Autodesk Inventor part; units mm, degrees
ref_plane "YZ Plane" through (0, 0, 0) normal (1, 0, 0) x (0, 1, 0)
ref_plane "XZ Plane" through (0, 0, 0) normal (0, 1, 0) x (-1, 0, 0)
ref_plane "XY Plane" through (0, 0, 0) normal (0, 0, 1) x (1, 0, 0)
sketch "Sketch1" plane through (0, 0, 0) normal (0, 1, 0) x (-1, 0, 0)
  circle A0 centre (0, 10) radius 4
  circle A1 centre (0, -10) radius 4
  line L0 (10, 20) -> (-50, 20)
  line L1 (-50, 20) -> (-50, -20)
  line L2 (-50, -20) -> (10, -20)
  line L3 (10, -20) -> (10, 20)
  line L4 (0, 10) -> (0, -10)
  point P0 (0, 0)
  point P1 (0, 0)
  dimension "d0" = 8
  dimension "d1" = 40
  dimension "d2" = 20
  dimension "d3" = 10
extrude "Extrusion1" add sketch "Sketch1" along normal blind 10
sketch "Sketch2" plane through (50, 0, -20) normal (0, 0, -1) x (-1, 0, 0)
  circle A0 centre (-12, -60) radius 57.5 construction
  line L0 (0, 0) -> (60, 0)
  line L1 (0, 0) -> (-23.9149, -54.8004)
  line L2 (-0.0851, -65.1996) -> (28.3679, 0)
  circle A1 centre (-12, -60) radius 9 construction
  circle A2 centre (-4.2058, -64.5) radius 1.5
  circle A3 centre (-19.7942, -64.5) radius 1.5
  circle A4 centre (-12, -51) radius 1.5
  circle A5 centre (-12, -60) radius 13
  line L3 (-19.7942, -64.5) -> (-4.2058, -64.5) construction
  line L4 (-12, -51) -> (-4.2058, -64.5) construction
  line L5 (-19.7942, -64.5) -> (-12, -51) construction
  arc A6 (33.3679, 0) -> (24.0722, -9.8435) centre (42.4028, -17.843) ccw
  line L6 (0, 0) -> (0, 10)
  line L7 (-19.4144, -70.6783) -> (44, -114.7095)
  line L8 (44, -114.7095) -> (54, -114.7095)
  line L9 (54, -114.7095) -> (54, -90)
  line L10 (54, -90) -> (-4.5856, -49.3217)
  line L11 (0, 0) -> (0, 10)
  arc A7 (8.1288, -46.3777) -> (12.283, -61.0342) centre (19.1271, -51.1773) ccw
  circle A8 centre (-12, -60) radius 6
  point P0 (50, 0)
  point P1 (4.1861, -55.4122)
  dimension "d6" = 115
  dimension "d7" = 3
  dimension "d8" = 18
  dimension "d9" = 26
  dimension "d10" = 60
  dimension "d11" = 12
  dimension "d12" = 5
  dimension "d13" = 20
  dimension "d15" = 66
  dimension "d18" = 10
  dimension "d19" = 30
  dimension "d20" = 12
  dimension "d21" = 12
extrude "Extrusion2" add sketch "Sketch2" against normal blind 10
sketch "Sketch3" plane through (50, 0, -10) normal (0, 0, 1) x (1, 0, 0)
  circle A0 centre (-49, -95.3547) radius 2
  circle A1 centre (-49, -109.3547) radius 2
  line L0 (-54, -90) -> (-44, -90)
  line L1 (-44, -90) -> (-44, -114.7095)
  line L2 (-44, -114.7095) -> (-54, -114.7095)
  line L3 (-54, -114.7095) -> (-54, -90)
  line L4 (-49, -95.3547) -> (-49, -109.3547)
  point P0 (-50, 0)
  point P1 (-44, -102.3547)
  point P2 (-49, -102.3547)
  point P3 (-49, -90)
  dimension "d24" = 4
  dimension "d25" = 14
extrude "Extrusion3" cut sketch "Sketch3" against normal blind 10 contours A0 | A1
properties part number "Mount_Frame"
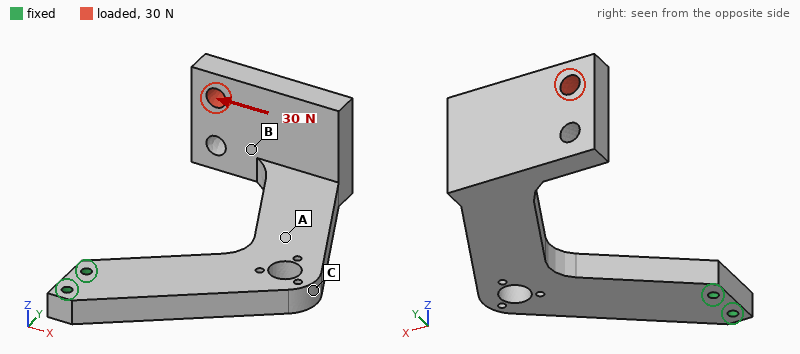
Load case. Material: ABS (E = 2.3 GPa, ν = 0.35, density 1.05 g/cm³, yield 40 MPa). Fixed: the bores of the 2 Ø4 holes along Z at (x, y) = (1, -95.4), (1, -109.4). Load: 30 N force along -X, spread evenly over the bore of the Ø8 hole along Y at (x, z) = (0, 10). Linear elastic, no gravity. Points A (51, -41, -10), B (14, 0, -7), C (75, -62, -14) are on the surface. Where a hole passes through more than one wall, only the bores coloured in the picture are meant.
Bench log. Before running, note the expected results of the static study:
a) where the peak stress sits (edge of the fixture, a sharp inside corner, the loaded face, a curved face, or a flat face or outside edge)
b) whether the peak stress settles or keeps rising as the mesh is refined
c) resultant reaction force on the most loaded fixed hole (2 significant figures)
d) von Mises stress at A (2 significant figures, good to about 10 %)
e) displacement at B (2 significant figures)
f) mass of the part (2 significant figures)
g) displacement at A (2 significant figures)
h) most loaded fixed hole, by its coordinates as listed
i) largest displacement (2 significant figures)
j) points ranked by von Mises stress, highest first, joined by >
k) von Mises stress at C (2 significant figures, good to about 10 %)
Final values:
edge of the fixture
keeps rising
210 N
2.2 MPa
0.84 mm
62 g
0.44 mm
(1, -95.4)
1.6 mm
A > C > B
0.89 MPa
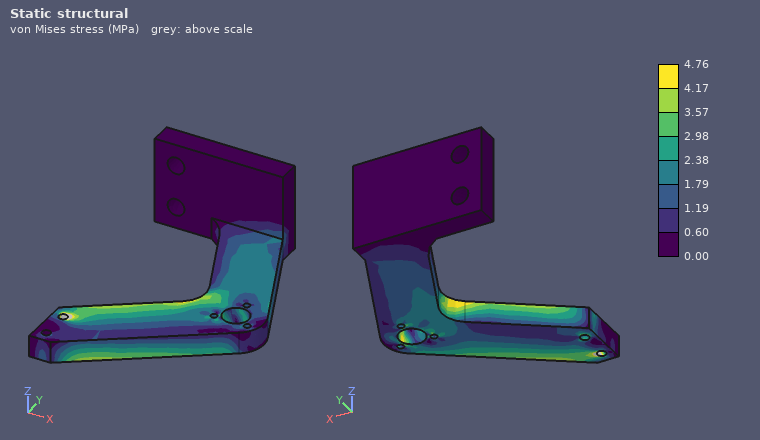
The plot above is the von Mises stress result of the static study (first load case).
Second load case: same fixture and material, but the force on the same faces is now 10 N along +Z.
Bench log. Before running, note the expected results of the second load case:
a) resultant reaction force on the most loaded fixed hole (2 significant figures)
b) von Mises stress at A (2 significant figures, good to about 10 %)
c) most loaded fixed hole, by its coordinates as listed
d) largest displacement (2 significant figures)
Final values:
44 N
1.6 MPa
(1, -95.4)
1.7 mm
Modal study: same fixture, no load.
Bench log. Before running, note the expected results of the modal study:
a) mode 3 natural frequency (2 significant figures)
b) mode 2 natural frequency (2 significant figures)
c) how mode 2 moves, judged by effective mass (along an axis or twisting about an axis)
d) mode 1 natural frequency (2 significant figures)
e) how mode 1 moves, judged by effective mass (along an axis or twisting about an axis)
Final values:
250 Hz
170 Hz
along X
81 Hz
along Z
